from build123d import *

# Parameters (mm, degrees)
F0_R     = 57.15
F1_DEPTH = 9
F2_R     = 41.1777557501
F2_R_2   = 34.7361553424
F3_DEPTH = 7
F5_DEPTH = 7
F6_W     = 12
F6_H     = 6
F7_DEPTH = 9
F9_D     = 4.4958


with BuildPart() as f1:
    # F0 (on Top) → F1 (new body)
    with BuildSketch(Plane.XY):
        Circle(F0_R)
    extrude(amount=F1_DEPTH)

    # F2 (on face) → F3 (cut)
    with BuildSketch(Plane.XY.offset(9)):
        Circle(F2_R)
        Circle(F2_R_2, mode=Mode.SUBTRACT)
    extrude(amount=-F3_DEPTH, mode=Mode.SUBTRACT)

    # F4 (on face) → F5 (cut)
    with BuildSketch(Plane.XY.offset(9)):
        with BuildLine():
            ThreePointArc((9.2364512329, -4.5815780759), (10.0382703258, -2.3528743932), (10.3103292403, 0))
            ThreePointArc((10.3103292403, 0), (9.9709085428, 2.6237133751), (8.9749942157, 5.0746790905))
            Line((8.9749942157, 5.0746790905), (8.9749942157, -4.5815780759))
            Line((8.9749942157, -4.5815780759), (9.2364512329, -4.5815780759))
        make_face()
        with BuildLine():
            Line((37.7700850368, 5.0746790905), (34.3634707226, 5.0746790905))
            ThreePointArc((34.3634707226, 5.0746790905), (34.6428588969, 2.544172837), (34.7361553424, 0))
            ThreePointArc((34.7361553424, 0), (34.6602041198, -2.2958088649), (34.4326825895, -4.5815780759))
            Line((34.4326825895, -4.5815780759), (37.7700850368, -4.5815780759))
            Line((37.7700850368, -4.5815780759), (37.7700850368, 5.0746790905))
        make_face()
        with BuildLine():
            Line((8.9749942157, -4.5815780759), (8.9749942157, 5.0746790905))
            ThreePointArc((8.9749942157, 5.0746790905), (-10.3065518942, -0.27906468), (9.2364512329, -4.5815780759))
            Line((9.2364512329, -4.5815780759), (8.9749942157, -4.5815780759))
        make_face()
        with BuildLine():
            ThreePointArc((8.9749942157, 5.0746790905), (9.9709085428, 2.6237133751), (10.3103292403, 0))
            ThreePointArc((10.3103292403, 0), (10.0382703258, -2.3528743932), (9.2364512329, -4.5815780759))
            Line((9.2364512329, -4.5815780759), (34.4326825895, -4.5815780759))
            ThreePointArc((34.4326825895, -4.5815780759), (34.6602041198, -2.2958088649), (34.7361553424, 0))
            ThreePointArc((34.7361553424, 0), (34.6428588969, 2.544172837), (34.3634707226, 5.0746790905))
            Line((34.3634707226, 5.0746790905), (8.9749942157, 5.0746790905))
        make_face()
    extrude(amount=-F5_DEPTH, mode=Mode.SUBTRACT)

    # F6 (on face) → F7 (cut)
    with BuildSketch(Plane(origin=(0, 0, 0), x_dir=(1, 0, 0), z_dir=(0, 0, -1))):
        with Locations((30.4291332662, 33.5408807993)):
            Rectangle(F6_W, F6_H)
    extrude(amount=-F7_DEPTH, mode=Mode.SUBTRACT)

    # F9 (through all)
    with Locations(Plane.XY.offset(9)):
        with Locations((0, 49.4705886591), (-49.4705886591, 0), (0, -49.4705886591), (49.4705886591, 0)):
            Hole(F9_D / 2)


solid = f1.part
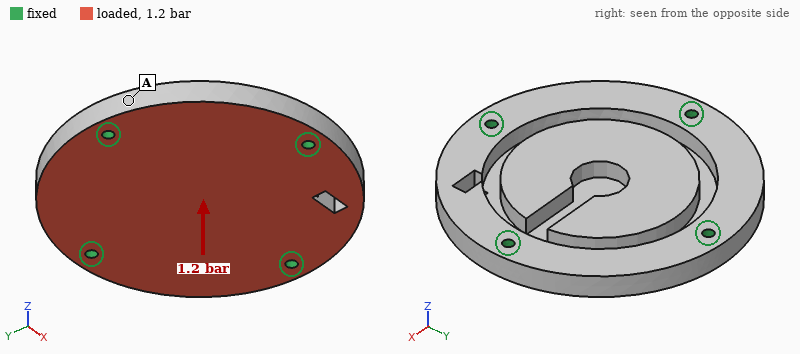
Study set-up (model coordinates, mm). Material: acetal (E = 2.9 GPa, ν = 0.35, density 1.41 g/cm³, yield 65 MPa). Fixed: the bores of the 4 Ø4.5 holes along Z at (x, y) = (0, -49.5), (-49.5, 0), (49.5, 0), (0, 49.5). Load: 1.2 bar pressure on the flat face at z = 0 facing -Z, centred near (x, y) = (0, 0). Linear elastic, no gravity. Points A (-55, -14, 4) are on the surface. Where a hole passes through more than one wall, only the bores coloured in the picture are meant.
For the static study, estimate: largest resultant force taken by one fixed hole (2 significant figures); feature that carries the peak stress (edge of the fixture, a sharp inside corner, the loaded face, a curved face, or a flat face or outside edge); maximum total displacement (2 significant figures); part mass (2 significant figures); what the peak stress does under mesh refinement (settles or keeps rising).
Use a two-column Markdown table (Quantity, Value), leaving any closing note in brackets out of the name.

| Quantity | Value |
|---|---|
| largest resultant force taken by one fixed hole | 320 N |
| feature that carries the peak stress | edge of the fixture |
| maximum total displacement | 0.30 mm |
| part mass | 110 g |
| what the peak stress does under mesh refinement | keeps rising |
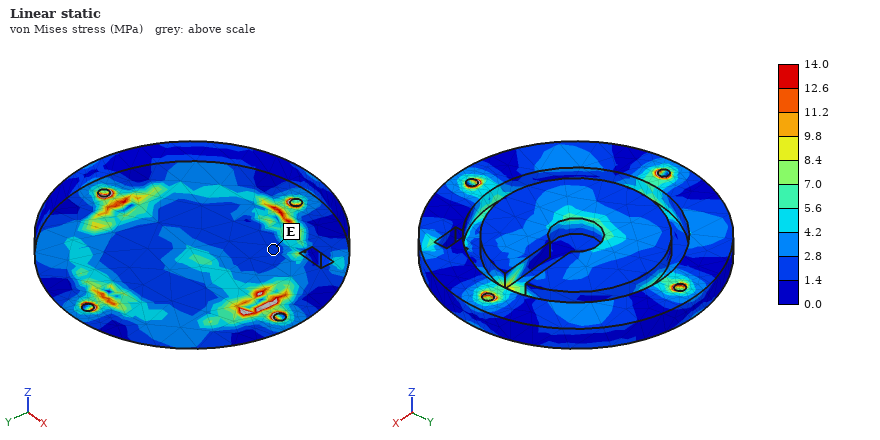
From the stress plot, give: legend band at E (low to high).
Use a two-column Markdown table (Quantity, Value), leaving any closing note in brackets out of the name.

| Quantity | Value |
|---|---|
| legend band at E | 1.4 to 2.8 MPa |
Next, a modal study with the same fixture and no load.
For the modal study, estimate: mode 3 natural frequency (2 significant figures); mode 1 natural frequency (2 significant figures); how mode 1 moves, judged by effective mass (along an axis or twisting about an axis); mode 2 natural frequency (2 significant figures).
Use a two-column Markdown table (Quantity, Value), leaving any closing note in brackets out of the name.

| Quantity | Value |
|---|---|
| mode 3 natural frequency | 1800 Hz |
| mode 1 natural frequency | 1300 Hz |
| how mode 1 moves, judged by effective mass | along Z |
| mode 2 natural frequency | 1800 Hz |
